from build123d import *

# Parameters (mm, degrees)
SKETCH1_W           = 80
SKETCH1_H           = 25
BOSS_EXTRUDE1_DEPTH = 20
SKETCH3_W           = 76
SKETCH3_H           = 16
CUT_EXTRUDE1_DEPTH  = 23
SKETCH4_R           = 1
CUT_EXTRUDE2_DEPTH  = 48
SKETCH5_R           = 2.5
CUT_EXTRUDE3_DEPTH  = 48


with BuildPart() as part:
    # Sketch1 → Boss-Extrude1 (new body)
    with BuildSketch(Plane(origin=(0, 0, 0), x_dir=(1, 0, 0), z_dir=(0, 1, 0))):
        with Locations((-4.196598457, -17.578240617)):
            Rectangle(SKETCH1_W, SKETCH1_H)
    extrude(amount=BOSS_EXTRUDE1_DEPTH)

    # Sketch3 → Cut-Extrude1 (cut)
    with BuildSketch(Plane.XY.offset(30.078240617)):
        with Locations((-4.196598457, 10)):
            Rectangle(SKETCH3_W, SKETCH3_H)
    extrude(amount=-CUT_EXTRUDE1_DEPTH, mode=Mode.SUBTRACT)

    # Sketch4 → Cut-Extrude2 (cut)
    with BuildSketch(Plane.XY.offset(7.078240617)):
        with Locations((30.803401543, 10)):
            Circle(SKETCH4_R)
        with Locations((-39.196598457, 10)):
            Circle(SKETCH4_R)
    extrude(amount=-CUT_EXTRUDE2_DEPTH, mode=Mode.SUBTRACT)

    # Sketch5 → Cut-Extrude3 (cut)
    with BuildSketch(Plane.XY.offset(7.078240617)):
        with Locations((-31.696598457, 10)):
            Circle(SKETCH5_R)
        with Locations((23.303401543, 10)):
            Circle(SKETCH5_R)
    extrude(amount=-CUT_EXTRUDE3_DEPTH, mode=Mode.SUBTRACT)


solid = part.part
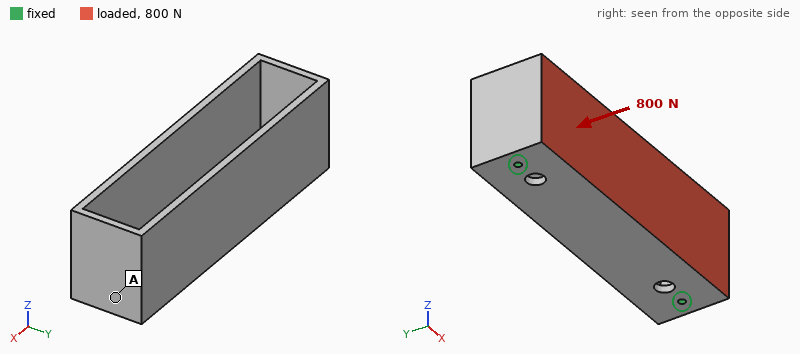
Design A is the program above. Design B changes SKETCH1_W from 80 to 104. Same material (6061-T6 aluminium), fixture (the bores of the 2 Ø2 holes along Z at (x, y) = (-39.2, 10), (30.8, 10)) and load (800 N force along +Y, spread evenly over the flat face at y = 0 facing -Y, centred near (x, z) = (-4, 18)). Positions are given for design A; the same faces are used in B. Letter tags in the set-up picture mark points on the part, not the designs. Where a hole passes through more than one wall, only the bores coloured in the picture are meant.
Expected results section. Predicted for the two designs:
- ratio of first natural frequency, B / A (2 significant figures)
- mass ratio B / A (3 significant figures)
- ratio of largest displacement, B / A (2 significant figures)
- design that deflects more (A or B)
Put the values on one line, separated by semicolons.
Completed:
0.74; 2.00; 0.81; A
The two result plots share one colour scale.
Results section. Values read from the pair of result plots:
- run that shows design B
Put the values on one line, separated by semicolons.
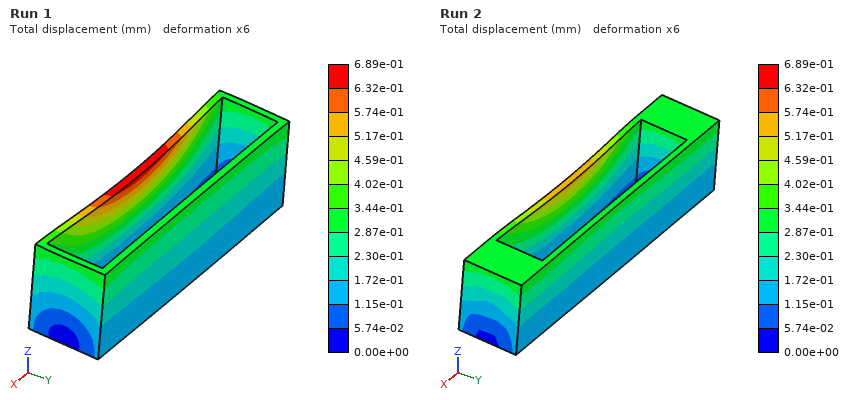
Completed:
Run 2
